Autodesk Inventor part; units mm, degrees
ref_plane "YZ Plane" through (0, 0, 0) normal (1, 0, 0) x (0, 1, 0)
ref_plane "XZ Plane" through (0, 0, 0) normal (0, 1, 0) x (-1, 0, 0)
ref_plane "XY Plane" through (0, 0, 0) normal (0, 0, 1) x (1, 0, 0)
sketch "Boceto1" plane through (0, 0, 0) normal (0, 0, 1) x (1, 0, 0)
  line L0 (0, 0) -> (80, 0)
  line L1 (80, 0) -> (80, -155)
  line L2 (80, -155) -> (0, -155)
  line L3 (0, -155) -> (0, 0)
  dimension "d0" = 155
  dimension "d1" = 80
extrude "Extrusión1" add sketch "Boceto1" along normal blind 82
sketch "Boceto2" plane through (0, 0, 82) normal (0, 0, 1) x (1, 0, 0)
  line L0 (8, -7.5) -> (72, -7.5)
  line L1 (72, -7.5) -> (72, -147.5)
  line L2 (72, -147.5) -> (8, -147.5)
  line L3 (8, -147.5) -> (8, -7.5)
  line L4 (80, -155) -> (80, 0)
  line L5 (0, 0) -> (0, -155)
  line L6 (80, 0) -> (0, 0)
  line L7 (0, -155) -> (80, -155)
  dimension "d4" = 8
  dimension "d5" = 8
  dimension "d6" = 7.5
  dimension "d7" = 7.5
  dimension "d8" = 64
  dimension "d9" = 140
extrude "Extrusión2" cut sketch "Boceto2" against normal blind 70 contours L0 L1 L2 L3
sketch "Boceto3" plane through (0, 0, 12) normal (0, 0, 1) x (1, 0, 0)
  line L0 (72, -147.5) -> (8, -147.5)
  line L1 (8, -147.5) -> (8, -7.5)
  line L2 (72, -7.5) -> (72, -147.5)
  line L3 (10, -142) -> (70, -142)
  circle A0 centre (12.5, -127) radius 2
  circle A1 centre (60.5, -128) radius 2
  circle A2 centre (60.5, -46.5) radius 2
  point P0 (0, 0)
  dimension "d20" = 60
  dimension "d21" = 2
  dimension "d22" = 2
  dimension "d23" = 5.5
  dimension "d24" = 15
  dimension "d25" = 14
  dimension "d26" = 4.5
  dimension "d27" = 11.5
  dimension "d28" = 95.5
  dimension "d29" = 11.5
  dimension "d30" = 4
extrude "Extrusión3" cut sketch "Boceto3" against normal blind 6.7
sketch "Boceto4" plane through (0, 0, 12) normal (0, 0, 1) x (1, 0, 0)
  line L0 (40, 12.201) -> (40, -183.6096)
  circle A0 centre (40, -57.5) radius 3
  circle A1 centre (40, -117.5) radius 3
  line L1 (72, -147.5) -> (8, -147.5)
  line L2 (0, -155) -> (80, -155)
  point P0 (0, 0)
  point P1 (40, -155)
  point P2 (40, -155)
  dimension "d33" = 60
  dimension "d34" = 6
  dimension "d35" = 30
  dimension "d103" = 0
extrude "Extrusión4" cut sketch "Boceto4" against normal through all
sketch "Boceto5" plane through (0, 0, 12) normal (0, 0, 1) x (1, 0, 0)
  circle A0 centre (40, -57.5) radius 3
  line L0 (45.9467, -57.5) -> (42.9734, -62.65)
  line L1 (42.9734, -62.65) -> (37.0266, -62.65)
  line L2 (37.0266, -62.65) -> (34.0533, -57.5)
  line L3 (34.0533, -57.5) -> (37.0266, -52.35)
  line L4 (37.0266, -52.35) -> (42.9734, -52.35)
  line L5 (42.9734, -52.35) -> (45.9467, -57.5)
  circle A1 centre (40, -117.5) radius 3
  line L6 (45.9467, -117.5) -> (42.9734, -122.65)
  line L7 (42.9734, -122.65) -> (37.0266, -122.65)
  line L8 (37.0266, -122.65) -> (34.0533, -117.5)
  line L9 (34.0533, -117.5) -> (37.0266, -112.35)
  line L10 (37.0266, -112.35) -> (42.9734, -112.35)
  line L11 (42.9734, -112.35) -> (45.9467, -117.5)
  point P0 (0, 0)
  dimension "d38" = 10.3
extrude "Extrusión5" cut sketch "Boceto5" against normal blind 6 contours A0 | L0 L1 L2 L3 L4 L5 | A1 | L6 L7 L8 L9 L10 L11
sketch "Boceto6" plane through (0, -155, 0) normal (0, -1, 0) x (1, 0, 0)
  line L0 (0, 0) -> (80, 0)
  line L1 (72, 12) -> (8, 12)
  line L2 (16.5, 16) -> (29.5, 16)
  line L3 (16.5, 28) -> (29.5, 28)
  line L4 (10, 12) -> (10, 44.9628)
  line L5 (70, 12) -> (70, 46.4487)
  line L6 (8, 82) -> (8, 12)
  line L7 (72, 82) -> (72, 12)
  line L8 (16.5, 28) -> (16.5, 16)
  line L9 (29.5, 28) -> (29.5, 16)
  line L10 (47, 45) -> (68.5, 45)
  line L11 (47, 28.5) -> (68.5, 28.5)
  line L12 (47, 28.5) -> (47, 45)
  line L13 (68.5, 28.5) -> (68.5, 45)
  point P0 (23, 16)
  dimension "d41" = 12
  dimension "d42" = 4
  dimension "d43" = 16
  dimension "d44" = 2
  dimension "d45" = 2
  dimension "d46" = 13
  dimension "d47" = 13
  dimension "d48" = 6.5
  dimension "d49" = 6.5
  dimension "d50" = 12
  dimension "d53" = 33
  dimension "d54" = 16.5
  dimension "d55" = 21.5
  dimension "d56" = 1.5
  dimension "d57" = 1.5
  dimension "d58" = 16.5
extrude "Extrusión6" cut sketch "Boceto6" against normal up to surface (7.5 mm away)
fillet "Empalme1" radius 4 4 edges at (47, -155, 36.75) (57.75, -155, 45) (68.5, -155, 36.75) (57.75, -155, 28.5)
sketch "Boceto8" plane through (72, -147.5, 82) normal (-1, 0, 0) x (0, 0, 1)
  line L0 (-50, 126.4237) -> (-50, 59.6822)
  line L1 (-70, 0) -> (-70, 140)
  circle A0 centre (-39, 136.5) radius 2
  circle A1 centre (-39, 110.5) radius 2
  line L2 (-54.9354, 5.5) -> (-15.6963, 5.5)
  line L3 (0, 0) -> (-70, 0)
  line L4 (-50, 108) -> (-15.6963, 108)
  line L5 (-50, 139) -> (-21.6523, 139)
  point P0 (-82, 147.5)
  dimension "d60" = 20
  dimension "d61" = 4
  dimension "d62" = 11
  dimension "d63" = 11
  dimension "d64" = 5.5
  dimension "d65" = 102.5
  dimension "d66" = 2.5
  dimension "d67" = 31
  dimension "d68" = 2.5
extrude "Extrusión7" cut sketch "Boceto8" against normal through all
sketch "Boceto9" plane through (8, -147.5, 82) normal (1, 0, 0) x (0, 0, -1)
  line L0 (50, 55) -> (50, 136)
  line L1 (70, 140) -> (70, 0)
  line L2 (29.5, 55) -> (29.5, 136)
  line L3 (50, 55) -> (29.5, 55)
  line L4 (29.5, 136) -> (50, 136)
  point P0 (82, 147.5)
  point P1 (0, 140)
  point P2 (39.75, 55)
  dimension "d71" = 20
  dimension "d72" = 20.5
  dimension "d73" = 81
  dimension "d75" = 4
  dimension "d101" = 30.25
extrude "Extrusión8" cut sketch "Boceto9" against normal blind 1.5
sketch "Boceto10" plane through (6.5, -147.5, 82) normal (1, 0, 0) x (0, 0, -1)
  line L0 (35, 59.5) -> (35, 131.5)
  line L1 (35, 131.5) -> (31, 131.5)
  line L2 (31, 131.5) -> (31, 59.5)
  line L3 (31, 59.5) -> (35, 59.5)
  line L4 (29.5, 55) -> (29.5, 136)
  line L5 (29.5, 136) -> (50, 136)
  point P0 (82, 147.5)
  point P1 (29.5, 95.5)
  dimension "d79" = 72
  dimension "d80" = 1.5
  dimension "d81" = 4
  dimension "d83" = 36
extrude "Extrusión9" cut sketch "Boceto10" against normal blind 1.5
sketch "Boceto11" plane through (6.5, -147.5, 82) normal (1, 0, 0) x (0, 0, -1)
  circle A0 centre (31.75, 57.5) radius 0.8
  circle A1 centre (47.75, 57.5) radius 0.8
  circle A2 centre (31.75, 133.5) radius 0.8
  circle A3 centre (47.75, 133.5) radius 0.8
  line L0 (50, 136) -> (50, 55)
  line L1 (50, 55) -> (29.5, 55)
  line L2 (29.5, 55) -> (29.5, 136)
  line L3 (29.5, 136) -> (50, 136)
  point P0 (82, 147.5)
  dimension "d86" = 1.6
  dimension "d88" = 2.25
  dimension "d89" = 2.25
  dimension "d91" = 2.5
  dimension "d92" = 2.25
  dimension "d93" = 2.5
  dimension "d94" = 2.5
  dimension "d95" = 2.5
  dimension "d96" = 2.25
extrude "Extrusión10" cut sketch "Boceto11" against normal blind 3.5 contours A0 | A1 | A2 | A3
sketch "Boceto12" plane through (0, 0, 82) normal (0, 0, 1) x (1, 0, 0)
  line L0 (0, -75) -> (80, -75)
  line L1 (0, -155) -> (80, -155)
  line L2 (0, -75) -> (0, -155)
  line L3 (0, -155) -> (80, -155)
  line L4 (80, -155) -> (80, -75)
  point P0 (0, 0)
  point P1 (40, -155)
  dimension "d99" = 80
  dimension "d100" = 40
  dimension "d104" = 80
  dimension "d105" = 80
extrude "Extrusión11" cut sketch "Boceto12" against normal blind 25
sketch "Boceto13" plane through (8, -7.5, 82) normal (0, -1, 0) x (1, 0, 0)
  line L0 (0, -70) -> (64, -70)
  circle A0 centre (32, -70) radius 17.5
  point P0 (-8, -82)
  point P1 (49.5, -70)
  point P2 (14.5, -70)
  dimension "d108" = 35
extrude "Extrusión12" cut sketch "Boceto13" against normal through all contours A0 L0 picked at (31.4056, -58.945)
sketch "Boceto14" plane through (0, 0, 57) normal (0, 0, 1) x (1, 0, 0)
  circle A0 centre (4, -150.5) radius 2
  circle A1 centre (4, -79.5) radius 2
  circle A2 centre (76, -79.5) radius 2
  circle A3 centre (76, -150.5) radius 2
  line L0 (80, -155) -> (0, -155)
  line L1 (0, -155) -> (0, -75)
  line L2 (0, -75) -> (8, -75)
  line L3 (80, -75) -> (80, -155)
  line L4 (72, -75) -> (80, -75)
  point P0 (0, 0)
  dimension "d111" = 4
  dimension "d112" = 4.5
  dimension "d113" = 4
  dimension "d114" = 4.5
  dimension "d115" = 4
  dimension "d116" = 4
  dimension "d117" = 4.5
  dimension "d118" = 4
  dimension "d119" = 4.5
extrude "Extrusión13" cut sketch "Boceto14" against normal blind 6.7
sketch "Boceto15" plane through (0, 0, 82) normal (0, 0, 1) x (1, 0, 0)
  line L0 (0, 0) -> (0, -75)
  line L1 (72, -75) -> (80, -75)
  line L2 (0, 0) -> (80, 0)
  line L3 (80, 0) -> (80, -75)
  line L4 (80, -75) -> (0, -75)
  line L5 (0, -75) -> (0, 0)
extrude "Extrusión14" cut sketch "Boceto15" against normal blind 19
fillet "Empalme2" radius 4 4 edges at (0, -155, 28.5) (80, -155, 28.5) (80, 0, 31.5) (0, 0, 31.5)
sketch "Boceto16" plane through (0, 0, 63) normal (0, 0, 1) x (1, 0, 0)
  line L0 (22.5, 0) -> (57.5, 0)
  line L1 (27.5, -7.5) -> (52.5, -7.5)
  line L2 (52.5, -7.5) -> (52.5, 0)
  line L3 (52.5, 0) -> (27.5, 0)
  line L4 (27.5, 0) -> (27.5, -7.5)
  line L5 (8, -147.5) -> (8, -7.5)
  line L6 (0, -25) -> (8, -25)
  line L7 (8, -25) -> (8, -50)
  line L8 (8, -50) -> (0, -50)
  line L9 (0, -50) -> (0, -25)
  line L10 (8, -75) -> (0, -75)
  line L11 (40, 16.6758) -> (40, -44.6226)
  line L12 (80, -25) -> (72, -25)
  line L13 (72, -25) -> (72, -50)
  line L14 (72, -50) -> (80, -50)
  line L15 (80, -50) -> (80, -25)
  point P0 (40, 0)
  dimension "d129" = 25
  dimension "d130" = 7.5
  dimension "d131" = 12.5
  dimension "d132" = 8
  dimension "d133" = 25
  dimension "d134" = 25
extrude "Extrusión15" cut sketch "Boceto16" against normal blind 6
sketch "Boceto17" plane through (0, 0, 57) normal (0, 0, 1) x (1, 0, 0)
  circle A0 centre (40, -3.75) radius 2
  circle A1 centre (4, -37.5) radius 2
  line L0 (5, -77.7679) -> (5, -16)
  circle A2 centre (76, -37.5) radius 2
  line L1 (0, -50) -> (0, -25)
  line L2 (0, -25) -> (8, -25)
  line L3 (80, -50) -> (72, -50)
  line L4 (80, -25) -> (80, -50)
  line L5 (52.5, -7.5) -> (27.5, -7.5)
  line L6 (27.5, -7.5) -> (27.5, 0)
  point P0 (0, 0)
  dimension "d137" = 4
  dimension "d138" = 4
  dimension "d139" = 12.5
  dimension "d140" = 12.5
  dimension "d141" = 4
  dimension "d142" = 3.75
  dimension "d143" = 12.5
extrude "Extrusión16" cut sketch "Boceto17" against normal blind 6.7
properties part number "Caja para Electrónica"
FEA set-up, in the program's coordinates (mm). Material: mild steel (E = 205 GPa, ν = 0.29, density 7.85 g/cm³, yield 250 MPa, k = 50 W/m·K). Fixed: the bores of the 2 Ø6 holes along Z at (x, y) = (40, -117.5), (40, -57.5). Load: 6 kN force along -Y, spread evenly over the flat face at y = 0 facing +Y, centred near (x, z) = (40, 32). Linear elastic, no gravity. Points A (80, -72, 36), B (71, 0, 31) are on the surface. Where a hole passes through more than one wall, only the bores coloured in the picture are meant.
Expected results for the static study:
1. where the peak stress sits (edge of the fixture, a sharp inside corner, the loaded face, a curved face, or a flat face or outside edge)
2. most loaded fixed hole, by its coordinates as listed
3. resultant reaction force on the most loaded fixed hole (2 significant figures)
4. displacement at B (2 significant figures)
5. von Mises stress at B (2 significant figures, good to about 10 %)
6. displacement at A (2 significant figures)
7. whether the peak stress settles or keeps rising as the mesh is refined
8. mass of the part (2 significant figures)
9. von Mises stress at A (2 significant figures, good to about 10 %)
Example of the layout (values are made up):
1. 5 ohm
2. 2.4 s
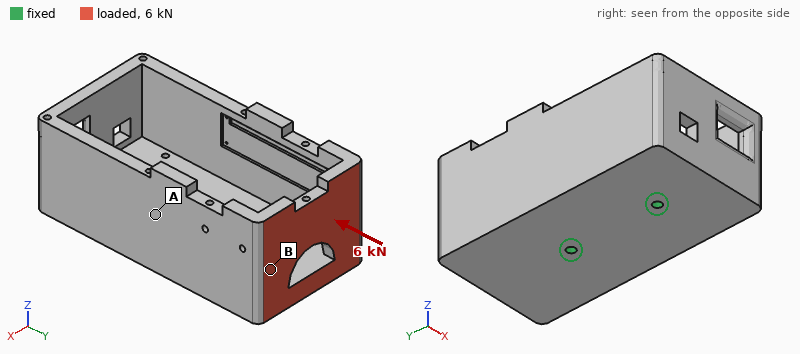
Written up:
1. edge of the fixture
2. (40, -57.5)
3. 4.2 kN
4. 24 µm
5. 25 MPa
6. 9.5 µm
7. keeps rising
8. 2.3 kg
9. 9.3 MPa
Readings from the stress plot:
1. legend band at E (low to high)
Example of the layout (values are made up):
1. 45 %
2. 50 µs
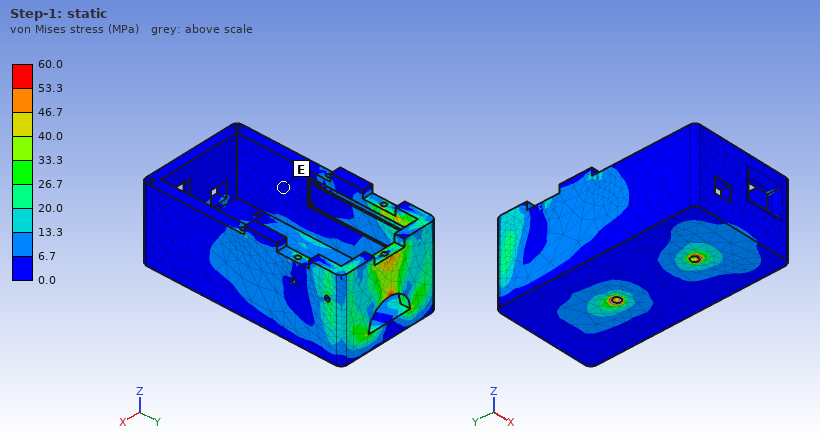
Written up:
1. 0.0 to 6.7 MPa
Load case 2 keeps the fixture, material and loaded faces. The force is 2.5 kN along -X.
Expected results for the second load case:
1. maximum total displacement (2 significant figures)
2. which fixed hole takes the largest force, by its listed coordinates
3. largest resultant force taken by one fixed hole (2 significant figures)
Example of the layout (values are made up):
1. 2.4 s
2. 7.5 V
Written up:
1. 0.12 mm
2. (40, -57.5)
3. 4.7 kN
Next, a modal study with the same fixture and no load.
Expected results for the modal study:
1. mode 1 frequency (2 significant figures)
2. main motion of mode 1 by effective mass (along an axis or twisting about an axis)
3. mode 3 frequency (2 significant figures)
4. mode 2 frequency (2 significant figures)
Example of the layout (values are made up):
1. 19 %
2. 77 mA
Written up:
1. 730 Hz
2. along X
3. 1700 Hz
4. 1600 Hz
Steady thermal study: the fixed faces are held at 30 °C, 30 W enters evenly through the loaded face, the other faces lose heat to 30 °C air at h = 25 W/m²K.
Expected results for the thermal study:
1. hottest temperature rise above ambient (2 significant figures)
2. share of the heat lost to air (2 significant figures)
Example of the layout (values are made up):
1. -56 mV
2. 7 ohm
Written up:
1. 34 K
2. 54 %
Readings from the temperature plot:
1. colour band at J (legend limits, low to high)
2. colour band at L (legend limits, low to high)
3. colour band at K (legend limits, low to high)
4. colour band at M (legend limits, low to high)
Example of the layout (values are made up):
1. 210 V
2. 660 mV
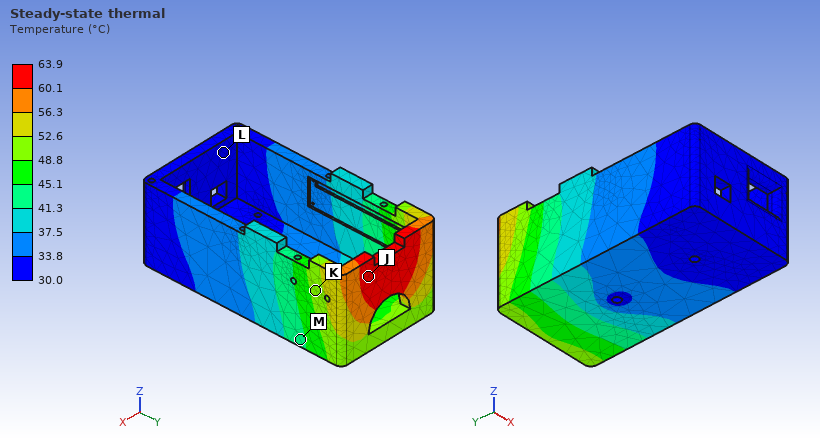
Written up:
1. 60.1 to 63.9 °C
2. 30.0 to 33.8 °C
3. 48.8 to 52.6 °C
4. 41.3 to 45.1 °C
